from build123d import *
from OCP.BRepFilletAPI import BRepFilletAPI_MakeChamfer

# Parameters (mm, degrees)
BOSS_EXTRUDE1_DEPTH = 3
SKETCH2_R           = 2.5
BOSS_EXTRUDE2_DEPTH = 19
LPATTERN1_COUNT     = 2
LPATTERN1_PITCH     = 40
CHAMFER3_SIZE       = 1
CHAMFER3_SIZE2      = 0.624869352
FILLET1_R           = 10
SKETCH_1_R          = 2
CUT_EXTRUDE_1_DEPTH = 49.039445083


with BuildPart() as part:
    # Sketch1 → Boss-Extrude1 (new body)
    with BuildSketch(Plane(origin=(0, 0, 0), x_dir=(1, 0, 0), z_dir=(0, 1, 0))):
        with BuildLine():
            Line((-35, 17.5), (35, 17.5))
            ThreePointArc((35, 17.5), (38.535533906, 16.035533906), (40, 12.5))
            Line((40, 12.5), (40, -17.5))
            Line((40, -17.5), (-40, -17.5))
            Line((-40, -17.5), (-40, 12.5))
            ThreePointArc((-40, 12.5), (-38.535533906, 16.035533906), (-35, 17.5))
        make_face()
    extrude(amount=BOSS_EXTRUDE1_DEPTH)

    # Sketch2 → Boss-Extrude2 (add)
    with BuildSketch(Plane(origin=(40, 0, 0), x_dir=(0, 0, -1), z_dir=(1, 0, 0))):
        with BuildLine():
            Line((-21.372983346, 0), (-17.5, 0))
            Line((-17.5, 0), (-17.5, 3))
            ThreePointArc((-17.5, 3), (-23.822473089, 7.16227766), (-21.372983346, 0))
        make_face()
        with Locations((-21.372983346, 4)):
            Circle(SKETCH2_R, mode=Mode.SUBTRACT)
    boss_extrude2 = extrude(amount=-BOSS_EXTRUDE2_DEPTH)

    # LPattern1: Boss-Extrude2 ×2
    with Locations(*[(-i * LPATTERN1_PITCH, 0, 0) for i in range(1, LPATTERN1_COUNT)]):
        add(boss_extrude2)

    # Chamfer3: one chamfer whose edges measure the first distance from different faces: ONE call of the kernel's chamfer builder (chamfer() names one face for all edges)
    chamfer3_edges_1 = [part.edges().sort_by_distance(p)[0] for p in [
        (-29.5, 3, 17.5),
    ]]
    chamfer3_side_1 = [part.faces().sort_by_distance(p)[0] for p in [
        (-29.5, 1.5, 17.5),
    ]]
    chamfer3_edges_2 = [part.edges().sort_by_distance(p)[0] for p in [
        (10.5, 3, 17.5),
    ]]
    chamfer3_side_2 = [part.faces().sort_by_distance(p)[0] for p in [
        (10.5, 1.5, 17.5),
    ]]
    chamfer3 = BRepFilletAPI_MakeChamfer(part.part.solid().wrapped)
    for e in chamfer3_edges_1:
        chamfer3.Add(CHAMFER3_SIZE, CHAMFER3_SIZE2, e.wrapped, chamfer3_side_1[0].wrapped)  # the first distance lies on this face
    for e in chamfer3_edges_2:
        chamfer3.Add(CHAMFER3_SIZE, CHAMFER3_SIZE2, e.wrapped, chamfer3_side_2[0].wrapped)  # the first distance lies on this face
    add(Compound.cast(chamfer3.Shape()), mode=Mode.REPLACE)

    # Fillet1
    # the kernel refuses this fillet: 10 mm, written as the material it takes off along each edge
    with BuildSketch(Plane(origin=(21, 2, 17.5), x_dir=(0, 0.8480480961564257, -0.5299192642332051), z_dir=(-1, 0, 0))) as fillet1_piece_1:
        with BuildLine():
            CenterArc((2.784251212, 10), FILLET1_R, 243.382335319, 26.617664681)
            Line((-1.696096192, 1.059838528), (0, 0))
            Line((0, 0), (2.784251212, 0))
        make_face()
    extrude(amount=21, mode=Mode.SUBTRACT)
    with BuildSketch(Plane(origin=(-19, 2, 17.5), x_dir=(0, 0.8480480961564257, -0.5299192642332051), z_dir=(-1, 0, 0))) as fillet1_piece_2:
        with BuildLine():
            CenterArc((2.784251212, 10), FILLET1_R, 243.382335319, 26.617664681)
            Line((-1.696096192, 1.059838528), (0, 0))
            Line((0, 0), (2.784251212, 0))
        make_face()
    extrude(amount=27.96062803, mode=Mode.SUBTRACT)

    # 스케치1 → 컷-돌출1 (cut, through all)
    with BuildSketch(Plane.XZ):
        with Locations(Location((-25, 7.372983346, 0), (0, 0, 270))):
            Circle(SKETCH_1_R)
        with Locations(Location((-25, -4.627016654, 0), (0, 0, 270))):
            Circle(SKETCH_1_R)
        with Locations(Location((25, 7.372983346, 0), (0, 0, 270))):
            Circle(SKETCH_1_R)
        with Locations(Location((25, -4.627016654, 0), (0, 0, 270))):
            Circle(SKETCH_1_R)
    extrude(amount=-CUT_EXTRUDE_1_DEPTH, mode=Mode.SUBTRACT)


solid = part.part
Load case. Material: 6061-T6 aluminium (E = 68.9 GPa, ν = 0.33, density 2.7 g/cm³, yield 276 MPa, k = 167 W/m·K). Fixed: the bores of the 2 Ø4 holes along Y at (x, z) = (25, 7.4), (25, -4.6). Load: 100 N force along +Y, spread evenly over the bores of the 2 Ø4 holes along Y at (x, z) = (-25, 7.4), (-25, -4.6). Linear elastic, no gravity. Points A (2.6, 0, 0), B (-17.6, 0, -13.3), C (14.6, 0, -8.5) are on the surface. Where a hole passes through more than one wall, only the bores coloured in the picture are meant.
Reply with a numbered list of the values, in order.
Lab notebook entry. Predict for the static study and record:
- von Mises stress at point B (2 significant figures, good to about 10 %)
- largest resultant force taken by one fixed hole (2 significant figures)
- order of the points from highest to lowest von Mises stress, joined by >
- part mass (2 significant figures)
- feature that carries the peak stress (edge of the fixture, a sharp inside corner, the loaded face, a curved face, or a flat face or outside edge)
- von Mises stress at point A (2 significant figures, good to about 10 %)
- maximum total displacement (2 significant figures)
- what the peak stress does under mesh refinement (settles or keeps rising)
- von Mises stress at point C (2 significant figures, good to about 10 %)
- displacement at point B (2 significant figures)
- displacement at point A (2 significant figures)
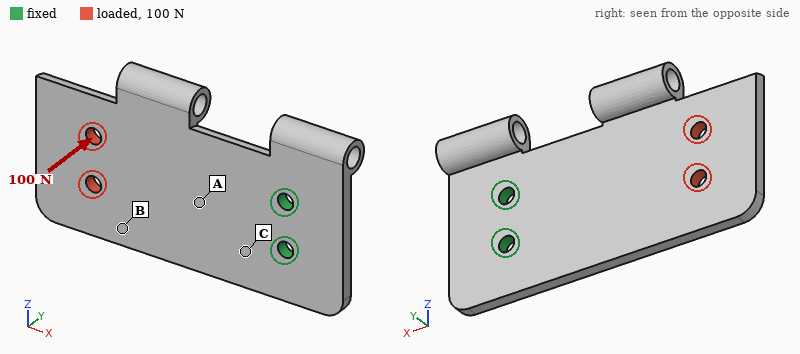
1. 14 MPa
2. 52 N
3. C > A > B
4. 26 g
5. edge of the fixture
6. 47 MPa
7. 1.0 mm
8. keeps rising
9. 68 MPa
10. 0.55 mm
11. 0.19 mm
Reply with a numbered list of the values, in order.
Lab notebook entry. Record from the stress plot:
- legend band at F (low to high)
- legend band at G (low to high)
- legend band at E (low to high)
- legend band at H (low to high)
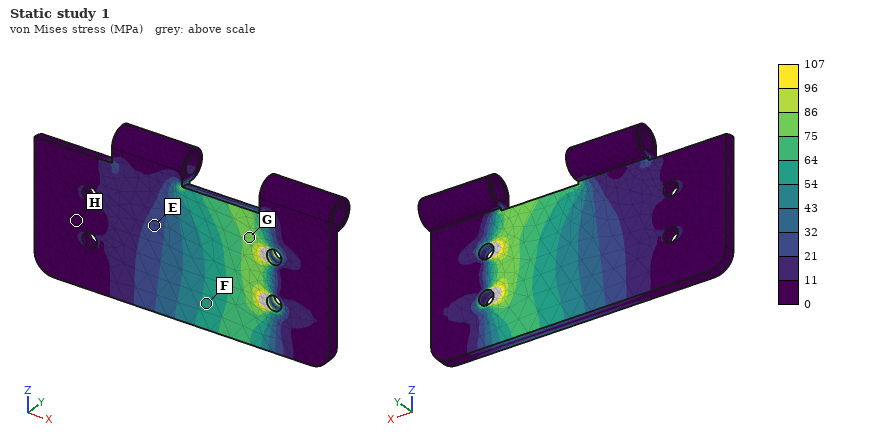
1. 54 to 64 MPa
2. 75 to 86 MPa
3. 21 to 32 MPa
4. 0 to 11 MPa
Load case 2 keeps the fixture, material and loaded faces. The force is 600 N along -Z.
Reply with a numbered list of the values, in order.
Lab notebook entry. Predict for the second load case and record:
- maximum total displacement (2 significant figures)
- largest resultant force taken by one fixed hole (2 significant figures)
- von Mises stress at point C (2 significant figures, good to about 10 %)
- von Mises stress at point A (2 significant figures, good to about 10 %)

1. 0.10 mm
2. 2.0 kN
3. 27 MPa
4. 17 MPa
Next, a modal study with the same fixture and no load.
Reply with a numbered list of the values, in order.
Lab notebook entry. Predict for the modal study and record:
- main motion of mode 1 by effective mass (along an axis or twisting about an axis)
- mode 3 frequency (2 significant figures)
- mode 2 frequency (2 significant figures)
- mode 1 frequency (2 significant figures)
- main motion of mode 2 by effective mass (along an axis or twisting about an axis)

1. along Y
2. 3600 Hz
3. 1900 Hz
4. 590 Hz
5. twisting about X
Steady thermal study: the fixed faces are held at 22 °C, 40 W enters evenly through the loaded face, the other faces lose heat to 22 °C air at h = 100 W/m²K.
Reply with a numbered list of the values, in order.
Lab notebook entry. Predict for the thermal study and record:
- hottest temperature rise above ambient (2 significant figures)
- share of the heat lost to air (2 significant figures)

1. 72 K
2. 55 %
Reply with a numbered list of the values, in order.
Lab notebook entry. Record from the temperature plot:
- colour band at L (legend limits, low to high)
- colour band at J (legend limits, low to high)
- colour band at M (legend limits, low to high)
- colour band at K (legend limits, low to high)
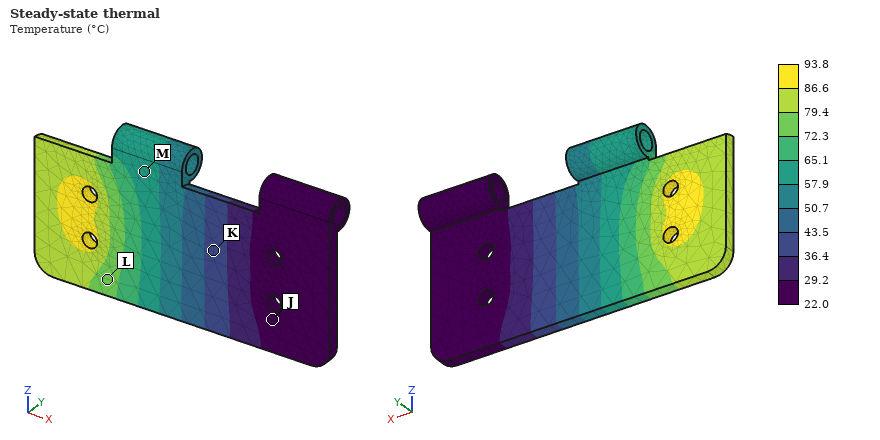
1. 72.3 to 79.4 °C
2. 22.0 to 29.2 °C
3. 57.9 to 65.1 °C
4. 36.4 to 43.5 °C
